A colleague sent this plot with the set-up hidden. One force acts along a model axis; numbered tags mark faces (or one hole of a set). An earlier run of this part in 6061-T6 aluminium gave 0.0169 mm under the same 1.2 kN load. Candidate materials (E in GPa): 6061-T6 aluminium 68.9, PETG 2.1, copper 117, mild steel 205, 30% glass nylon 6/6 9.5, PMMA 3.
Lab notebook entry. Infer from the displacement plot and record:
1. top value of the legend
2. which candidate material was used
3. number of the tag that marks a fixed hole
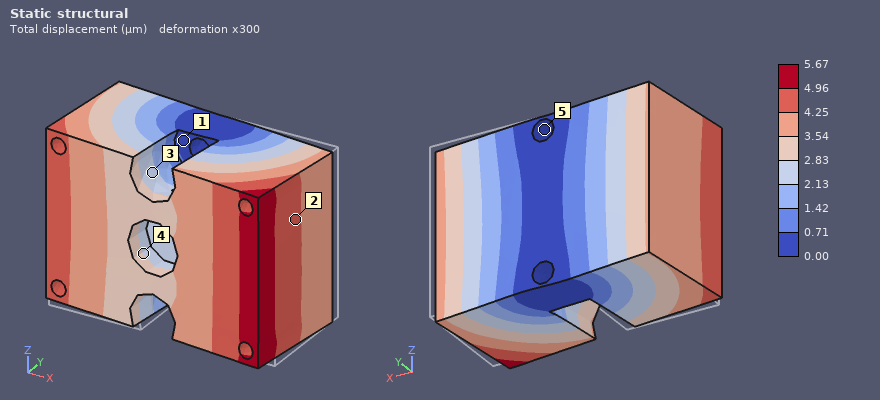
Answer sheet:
5.67 µm
mild steel
5
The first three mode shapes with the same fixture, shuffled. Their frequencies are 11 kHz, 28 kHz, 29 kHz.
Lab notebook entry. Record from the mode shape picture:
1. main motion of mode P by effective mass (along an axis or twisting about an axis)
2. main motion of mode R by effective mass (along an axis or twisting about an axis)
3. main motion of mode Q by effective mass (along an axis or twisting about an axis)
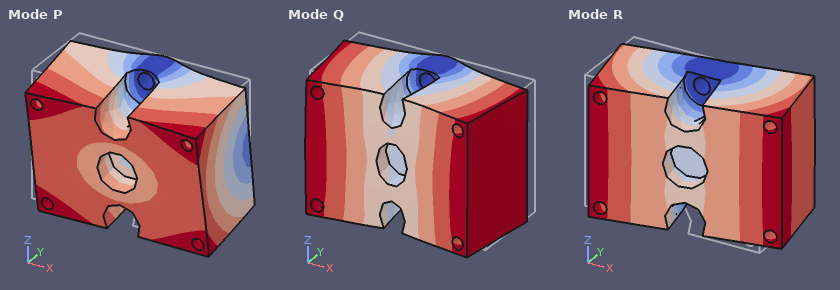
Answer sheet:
along Z
along X
along Y
